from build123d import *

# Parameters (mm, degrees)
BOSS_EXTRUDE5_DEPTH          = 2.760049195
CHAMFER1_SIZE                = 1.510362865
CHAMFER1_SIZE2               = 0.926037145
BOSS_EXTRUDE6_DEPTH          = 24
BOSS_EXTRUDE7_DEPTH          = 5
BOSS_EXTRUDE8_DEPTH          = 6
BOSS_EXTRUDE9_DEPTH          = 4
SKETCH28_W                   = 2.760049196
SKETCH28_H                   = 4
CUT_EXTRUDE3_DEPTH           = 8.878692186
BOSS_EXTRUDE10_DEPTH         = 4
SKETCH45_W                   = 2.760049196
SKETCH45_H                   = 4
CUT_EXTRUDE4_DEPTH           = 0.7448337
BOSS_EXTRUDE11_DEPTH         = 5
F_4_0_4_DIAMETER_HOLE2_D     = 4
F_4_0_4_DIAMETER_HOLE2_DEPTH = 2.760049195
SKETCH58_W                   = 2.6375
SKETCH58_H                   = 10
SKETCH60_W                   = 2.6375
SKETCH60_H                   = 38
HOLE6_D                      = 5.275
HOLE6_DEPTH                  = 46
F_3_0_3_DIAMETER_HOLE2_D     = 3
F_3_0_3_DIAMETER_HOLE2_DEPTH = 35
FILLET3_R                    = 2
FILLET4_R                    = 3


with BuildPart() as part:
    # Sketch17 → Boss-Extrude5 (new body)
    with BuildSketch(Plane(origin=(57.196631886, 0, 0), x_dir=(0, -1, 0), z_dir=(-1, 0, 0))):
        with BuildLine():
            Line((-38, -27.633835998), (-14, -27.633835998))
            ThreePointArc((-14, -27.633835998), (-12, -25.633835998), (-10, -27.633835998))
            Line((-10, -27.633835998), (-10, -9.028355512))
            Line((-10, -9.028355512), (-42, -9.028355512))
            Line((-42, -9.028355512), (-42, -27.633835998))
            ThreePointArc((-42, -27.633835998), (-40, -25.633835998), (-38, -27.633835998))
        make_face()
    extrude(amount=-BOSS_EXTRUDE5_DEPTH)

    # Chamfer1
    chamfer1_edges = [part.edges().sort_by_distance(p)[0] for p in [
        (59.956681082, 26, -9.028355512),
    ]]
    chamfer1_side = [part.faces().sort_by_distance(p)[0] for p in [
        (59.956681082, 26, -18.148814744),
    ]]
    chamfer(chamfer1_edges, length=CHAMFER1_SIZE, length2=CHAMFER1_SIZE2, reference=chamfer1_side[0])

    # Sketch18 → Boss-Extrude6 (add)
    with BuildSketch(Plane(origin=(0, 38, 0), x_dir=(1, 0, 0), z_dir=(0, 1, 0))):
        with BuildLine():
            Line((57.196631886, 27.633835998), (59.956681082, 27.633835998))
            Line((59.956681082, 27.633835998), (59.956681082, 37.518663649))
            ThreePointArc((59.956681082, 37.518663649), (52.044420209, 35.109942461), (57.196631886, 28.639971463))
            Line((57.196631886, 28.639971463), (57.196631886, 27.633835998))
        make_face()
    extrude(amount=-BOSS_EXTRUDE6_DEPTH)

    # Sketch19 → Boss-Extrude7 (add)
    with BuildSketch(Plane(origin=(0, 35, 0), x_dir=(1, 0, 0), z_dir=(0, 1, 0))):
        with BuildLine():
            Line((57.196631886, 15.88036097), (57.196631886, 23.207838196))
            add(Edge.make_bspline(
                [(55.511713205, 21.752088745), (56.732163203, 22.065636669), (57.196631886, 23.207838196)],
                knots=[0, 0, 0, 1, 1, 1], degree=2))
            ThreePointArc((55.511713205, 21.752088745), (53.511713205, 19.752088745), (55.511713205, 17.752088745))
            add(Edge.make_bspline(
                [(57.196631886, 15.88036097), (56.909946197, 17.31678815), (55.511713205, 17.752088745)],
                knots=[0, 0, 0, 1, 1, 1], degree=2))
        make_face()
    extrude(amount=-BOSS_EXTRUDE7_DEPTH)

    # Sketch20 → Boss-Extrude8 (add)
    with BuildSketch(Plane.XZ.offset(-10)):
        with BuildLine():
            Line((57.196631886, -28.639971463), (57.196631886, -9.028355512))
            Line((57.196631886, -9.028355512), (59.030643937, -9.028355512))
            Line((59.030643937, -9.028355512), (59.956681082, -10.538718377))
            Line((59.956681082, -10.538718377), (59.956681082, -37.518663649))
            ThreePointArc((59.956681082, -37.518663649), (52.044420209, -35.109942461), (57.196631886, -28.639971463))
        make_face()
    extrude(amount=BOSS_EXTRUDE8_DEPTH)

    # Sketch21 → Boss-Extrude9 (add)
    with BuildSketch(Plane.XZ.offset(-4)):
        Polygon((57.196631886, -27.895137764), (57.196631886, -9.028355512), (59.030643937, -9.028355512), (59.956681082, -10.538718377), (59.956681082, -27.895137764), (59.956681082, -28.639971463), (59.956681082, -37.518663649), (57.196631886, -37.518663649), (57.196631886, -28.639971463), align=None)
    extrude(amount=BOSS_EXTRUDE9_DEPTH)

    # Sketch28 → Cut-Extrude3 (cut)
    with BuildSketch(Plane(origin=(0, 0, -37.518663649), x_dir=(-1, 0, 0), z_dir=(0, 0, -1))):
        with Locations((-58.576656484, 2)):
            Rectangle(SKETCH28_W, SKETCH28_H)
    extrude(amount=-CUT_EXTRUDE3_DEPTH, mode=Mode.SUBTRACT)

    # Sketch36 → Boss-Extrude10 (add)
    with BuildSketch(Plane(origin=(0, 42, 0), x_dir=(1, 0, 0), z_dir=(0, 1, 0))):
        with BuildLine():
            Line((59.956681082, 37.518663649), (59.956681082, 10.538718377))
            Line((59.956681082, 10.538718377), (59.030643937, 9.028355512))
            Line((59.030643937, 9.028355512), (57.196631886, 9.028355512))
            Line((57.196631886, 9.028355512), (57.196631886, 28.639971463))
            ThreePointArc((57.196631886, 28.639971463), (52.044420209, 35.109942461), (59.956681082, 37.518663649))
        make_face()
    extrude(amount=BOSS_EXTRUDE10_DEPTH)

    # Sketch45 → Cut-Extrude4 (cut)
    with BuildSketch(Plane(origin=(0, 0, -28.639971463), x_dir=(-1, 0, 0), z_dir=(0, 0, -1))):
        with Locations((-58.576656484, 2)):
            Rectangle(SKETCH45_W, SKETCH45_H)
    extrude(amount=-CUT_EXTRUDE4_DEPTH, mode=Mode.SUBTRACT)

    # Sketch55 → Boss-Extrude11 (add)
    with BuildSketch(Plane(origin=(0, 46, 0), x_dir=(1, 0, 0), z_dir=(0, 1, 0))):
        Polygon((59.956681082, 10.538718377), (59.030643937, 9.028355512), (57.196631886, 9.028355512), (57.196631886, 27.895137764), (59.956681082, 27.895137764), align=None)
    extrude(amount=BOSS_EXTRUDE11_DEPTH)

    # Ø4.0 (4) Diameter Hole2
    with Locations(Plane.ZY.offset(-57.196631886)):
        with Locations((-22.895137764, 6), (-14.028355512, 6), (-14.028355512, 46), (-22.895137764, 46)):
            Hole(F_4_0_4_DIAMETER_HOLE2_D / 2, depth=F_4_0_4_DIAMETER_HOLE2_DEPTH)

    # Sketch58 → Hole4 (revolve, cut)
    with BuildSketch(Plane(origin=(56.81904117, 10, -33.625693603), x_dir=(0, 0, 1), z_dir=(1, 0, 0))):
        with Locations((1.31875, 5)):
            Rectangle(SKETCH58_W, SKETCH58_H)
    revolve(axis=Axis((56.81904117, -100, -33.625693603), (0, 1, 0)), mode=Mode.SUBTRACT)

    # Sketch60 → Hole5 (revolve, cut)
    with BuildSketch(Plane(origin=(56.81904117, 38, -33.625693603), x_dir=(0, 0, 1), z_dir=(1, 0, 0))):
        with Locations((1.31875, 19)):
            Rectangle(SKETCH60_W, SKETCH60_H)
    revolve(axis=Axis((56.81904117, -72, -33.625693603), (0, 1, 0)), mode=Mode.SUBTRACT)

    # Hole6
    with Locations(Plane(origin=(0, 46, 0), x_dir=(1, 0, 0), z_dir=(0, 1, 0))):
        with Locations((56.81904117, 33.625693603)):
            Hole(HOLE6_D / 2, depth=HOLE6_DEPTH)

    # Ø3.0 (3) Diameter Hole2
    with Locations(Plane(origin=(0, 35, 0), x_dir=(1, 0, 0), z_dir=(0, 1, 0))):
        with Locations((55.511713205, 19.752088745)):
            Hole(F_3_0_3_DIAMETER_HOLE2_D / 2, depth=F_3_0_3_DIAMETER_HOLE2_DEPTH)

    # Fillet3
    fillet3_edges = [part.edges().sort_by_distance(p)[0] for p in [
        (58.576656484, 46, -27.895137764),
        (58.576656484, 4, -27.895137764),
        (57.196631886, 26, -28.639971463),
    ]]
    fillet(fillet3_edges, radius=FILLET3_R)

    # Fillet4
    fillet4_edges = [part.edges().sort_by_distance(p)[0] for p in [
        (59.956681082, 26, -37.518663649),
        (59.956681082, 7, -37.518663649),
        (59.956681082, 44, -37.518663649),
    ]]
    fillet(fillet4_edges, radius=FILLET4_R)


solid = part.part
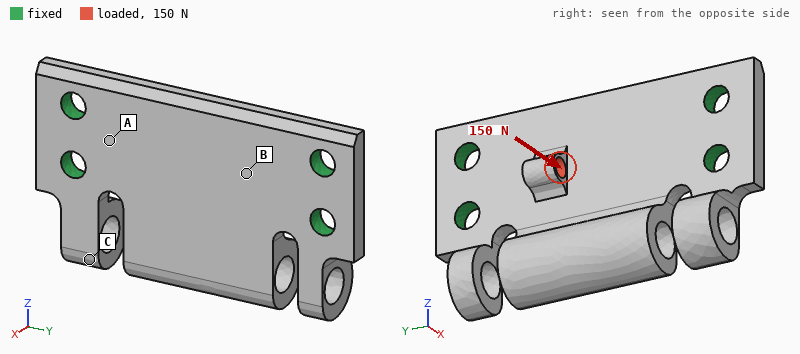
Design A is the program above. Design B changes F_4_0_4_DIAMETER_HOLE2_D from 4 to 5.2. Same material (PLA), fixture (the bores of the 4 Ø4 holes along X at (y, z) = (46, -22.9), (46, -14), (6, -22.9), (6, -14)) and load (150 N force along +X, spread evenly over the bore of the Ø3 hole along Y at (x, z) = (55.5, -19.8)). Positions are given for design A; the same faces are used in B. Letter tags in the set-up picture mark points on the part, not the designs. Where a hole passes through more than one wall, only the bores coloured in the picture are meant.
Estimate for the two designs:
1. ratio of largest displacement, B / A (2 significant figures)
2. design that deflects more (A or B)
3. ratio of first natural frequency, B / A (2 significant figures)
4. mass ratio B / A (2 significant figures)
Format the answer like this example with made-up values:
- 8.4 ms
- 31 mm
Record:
- 0.89
- A
- 1.0
- 0.98
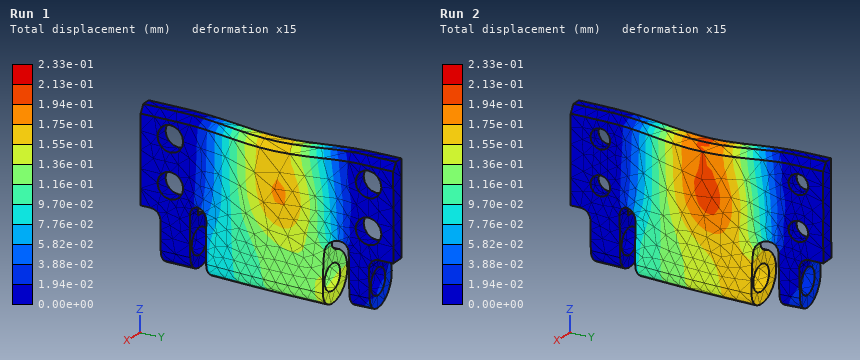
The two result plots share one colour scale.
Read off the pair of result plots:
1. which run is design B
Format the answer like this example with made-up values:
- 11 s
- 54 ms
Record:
- Run 1
